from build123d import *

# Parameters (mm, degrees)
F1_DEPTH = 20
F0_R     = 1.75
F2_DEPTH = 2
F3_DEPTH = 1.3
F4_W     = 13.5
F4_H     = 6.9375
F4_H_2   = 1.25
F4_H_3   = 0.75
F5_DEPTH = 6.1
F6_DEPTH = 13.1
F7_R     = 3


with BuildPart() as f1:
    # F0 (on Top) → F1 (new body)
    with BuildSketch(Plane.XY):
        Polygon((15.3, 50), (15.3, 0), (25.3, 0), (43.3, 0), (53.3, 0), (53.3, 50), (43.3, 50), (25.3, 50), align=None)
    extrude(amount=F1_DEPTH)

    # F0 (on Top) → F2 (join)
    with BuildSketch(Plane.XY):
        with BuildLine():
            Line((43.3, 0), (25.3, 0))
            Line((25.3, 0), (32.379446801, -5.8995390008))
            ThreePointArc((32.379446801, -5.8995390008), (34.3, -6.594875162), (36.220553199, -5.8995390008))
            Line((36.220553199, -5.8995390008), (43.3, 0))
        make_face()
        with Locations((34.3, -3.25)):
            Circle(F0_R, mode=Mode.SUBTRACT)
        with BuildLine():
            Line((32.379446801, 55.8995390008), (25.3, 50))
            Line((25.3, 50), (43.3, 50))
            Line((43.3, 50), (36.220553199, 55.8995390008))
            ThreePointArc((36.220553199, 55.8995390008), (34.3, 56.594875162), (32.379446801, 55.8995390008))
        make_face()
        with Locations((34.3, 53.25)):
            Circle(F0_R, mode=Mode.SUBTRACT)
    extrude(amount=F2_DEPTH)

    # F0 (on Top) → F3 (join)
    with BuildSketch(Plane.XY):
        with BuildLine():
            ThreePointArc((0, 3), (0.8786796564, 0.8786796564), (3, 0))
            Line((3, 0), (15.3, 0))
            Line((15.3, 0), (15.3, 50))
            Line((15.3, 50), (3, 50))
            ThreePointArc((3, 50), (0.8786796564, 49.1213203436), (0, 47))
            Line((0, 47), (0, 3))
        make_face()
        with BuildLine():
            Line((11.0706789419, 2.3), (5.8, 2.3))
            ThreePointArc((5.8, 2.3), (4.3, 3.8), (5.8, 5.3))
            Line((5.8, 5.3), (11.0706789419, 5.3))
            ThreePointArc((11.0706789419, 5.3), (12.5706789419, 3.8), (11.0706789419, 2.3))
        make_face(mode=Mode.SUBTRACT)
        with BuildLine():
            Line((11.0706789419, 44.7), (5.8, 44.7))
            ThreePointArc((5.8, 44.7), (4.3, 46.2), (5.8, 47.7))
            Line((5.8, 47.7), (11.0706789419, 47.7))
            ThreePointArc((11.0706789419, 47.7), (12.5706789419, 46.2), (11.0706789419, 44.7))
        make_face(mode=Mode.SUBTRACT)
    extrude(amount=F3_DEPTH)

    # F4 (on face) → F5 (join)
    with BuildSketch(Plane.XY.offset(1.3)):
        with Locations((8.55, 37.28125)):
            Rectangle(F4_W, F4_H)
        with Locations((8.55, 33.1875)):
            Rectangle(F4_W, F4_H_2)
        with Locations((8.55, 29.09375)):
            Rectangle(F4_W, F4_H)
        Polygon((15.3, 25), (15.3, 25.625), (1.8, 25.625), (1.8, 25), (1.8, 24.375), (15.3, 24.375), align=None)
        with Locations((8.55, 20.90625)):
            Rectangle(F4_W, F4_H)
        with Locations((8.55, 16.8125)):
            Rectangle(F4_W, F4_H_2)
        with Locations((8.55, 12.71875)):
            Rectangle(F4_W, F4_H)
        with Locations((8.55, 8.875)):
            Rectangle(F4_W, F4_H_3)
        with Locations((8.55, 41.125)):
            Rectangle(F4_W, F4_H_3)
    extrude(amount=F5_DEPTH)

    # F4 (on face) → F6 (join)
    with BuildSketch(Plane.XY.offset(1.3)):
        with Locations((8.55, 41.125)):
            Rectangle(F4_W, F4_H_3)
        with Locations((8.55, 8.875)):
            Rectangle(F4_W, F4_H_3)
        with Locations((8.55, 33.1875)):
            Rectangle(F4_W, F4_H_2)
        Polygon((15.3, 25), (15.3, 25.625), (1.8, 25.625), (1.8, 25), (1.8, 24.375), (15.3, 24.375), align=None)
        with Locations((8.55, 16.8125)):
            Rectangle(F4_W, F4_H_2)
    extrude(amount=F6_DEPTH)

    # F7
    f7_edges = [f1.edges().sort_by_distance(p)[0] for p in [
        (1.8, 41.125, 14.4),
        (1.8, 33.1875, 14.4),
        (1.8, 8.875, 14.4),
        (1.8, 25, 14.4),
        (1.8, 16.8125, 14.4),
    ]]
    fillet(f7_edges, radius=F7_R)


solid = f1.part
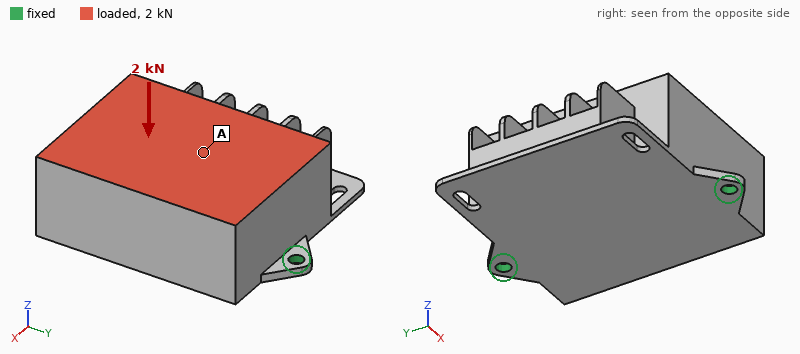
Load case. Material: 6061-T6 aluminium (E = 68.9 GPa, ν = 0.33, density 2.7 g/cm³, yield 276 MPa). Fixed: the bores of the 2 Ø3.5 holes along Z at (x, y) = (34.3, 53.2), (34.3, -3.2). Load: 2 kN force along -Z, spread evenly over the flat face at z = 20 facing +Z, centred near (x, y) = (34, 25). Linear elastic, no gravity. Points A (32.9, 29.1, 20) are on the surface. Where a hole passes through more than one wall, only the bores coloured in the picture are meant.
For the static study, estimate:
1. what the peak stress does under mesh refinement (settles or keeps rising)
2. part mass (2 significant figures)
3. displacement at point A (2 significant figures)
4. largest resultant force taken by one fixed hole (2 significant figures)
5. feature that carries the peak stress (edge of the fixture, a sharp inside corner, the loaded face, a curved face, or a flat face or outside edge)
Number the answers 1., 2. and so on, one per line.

1. keeps rising
2. 110 g
3. 18 µm
4. 1.1 kN
5. edge of the fixture
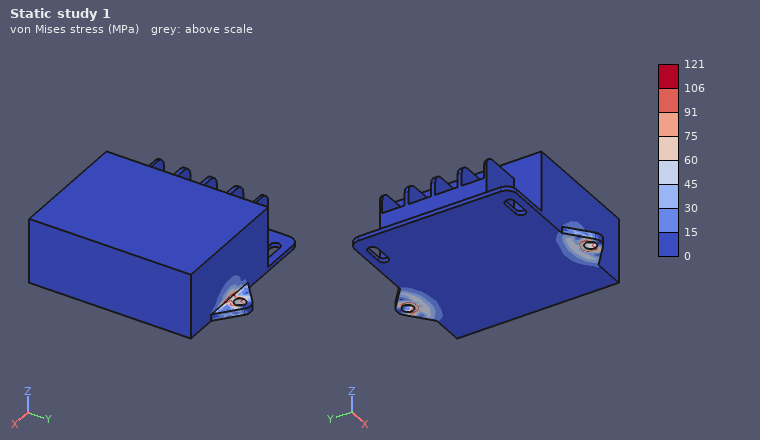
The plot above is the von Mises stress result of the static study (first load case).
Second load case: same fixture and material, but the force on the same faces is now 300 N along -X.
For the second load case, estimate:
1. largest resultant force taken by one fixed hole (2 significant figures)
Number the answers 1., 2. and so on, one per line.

1. 150 N
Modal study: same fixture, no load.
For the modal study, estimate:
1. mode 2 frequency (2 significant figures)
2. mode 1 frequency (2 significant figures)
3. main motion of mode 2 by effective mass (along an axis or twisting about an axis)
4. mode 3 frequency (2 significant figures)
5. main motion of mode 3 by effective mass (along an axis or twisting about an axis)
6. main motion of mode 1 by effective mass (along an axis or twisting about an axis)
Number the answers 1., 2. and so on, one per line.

1. 5100 Hz
2. 820 Hz
3. along Z
4. 7500 Hz
5. along Y
6. along X
